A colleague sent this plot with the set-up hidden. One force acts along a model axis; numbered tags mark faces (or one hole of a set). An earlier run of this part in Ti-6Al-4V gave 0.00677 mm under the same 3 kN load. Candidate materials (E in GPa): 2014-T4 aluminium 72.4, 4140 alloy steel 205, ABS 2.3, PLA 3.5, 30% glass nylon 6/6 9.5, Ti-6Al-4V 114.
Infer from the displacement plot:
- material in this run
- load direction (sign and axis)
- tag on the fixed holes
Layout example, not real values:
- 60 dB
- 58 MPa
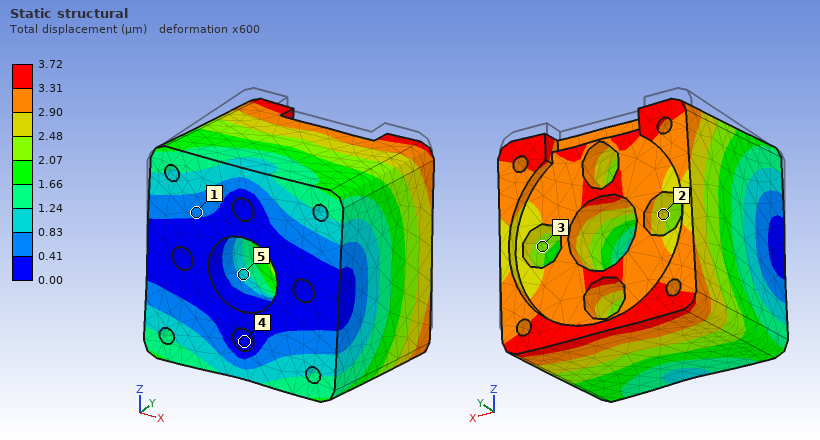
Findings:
- 4140 alloy steel
- -Z
- 4
